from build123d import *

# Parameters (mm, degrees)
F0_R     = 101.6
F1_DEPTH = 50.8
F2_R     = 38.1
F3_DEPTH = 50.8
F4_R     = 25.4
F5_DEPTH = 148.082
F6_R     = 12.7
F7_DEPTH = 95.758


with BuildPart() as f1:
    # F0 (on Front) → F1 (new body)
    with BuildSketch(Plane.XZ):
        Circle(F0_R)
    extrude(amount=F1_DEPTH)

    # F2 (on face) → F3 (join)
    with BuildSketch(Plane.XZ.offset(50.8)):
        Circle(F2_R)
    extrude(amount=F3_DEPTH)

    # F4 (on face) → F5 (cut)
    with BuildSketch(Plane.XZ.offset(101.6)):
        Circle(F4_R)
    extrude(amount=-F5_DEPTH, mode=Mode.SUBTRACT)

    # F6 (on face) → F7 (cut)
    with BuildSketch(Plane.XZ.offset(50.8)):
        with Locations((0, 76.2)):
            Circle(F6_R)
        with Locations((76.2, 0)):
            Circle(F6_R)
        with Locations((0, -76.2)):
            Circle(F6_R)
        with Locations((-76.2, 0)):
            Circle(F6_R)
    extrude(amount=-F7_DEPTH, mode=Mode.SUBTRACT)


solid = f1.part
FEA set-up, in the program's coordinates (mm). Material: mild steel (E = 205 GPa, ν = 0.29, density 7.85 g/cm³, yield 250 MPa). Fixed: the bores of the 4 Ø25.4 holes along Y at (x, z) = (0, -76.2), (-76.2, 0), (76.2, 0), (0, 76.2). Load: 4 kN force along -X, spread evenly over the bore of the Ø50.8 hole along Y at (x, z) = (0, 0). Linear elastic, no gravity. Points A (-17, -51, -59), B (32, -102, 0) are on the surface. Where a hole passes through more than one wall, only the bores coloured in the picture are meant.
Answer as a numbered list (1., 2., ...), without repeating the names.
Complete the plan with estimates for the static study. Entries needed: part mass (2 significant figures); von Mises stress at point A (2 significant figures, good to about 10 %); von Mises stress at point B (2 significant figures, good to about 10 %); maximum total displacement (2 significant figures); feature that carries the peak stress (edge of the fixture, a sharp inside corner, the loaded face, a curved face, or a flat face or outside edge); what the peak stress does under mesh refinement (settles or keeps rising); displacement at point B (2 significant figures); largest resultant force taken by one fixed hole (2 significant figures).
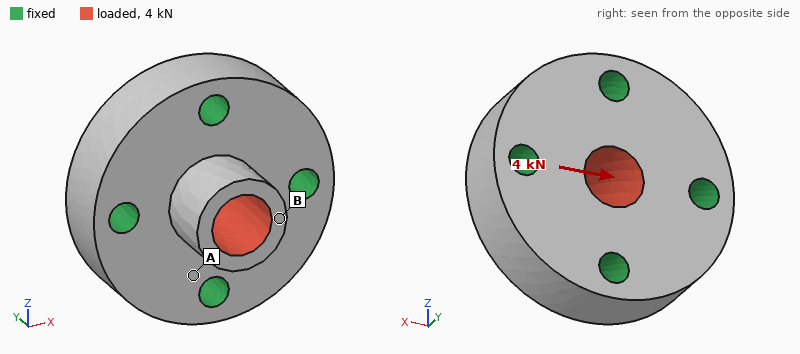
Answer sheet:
1. 12 kg
2. 0.35 MPa
3. 0.94 MPa
4. 1.1 µm
5. a sharp inside corner
6. keeps rising
7. 1.1 µm
8. 1.5 kN
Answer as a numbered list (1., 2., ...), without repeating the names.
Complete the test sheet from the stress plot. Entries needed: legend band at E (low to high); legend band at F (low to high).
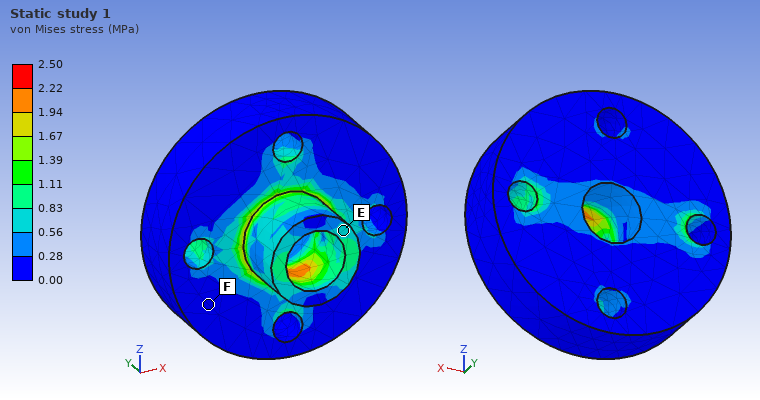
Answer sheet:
1. 0.56 to 0.83 MPa
2. 0.00 to 0.28 MPa
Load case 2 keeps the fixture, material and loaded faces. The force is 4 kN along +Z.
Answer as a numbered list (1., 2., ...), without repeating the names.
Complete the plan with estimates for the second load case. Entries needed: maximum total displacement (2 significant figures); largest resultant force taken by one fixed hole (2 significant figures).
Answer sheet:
1. 1.1 µm
2. 1.5 kN
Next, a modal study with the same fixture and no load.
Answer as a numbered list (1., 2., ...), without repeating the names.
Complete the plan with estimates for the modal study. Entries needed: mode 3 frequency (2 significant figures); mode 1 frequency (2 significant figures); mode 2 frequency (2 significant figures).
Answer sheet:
1. 9900 Hz
2. 8000 Hz
3. 8000 Hz
